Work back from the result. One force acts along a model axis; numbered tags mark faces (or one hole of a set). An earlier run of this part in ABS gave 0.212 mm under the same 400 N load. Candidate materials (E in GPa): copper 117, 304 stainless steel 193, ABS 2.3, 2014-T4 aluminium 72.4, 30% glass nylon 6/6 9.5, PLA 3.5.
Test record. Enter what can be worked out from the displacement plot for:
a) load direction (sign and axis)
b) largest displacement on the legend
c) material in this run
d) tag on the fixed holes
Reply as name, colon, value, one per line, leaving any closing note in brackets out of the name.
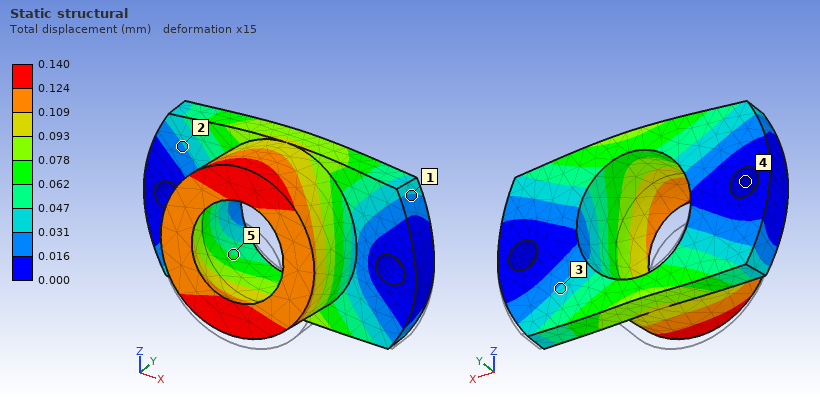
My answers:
load direction: +Z
largest displacement on the legend: 0.140 mm
material in this run: PLA
tag on the fixed holes: 4
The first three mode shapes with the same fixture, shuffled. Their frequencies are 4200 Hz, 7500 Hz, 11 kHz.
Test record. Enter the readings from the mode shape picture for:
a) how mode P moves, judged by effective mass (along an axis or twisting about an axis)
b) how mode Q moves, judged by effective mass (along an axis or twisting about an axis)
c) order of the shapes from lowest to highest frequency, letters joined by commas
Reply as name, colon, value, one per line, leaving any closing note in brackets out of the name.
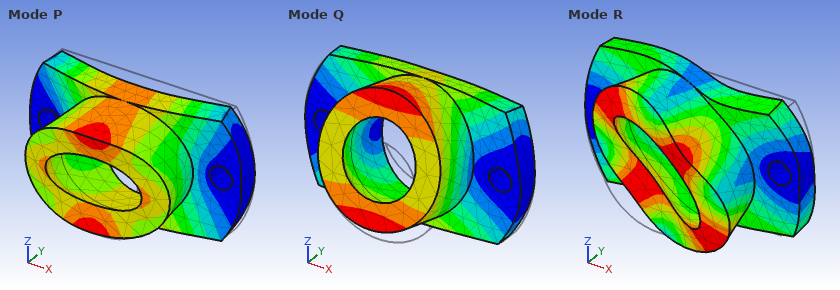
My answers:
how mode P moves, judged by effective mass: along Y
how mode Q moves, judged by effective mass: along Z
order of the shapes from lowest to highest frequency, letters joined by commas: Q, P, R
